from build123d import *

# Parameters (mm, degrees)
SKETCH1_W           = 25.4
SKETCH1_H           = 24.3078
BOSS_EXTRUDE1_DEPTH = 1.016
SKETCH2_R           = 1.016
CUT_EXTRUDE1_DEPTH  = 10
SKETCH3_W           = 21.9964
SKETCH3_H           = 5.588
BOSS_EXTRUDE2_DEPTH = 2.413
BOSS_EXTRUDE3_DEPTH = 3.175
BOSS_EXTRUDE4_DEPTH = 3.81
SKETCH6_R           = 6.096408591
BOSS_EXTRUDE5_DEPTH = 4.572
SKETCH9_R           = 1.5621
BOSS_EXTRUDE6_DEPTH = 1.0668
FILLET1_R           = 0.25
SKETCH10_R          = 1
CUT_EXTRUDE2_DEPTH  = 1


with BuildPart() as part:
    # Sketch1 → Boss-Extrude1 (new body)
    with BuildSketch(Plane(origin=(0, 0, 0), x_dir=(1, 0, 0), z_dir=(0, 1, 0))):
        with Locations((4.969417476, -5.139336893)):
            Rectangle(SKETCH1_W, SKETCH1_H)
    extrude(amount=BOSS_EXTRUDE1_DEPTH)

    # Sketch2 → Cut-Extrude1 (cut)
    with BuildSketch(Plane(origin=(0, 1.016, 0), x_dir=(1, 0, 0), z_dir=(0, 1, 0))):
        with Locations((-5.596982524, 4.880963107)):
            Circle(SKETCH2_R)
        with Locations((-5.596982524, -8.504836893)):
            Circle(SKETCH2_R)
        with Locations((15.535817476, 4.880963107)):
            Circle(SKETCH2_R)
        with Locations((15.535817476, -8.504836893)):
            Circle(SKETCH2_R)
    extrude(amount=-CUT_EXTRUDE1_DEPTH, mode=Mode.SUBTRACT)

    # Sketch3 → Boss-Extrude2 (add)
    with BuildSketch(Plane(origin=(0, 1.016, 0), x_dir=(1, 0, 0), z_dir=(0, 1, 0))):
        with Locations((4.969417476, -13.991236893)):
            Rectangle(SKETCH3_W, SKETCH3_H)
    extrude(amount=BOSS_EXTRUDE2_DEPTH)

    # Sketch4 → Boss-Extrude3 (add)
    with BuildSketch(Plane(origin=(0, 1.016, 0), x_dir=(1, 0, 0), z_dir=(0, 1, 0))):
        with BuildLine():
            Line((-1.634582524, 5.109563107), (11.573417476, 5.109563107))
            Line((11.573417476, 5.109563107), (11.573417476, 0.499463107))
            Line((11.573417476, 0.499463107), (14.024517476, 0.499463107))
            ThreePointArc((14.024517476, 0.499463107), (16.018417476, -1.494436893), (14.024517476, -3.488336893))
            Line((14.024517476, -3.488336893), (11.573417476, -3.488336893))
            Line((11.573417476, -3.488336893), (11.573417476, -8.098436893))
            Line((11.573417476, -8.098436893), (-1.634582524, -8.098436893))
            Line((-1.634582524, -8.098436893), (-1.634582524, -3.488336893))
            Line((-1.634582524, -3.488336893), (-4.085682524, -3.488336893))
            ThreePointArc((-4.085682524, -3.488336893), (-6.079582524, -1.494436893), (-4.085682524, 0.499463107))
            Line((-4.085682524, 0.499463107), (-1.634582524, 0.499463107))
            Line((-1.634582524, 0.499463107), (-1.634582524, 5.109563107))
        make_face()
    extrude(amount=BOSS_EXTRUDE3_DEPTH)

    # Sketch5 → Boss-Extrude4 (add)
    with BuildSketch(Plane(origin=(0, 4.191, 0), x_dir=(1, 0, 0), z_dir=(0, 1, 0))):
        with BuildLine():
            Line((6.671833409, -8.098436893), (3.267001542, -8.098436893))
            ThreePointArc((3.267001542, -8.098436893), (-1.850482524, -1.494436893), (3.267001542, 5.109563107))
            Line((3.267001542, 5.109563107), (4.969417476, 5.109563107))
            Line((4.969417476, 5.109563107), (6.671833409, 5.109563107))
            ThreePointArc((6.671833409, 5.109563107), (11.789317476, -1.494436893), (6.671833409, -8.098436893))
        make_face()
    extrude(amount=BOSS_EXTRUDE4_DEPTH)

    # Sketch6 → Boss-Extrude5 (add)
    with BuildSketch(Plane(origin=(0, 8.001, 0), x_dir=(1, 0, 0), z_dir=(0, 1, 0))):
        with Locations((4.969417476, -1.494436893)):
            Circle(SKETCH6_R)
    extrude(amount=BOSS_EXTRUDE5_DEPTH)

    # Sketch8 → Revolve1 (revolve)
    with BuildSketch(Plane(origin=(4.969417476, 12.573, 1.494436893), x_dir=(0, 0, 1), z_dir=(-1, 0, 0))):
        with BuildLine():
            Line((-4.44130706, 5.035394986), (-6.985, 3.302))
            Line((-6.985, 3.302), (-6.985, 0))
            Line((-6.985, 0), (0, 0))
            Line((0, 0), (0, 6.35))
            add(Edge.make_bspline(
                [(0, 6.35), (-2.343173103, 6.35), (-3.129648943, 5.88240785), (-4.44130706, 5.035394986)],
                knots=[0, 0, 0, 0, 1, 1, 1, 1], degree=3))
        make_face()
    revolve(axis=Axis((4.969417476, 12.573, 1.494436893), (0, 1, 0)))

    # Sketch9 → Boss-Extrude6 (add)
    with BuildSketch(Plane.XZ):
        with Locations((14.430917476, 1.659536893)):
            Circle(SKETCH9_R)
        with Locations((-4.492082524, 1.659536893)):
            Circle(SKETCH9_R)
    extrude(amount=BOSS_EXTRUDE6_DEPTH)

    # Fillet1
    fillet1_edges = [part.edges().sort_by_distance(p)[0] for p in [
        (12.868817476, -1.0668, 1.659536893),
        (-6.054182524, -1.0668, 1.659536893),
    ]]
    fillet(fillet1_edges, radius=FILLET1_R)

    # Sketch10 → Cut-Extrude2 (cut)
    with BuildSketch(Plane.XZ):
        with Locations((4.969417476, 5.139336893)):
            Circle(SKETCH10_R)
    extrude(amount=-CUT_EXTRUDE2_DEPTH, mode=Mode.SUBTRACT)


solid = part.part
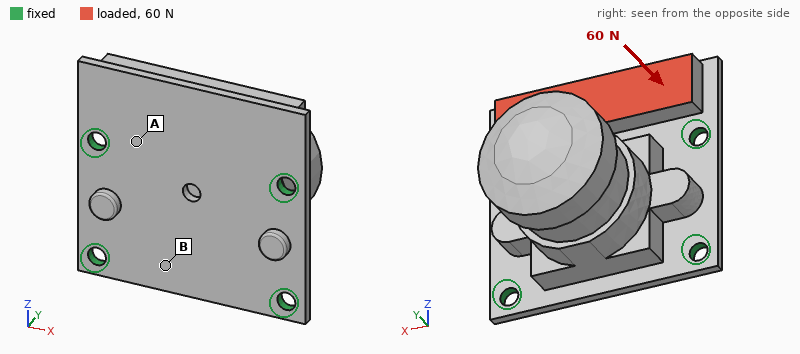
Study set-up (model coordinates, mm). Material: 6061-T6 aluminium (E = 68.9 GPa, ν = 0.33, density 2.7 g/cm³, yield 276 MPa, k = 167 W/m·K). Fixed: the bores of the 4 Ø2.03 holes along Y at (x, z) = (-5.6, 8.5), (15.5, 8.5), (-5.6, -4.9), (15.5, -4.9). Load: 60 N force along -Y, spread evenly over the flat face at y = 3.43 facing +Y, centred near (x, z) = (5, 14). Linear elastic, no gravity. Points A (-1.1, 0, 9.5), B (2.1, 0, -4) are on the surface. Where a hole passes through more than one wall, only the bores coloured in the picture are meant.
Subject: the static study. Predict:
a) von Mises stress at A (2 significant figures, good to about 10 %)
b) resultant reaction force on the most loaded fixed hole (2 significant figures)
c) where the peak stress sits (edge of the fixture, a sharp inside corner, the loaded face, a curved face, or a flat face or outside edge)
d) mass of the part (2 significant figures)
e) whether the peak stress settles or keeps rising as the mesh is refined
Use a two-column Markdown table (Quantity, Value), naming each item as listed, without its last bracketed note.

| Quantity | Value |
|---|---|
| von Mises stress at A | 36 MPa |
| resultant reaction force on the most loaded fixed hole | 41 N |
| where the peak stress sits | edge of the fixture |
| mass of the part | 9.2 g |
| whether the peak stress settles or keeps rising as the mesh is refined | keeps rising |
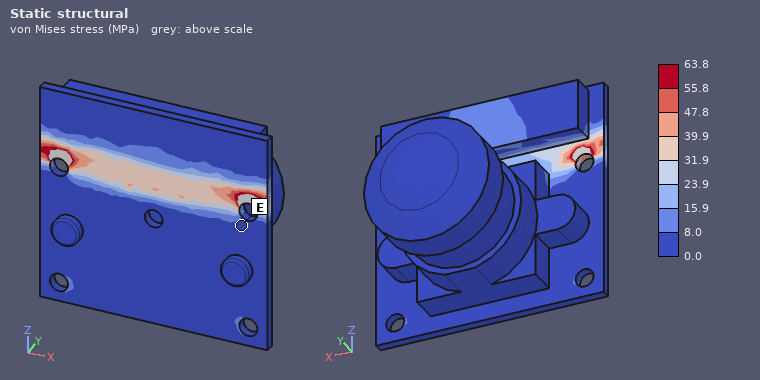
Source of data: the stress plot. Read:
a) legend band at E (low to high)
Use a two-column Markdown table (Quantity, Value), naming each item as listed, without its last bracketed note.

| Quantity | Value |
|---|---|
| legend band at E | 0.0 to 8.0 MPa |
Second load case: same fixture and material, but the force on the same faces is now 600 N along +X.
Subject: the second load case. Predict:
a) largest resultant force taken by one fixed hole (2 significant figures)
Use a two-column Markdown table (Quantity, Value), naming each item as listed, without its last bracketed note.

| Quantity | Value |
|---|---|
| largest resultant force taken by one fixed hole | 310 N |
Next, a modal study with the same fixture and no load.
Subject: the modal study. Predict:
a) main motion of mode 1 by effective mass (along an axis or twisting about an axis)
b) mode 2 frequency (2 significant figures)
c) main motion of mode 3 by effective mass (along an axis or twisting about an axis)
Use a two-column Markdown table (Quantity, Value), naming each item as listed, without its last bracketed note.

| Quantity | Value |
|---|---|
| main motion of mode 1 by effective mass | along Z |
| mode 2 frequency | 7100 Hz |
| main motion of mode 3 by effective mass | along X |
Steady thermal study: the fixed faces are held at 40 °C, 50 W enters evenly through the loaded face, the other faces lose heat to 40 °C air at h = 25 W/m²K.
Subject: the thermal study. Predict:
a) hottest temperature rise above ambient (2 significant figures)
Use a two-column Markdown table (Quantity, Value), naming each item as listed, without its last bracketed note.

| Quantity | Value |
|---|---|
| hottest temperature rise above ambient | 75 K |
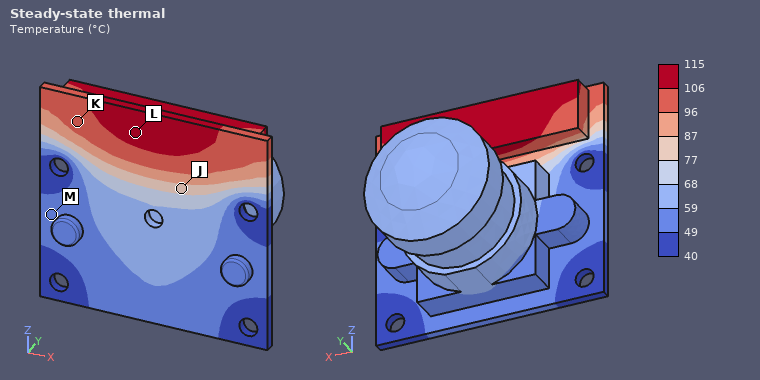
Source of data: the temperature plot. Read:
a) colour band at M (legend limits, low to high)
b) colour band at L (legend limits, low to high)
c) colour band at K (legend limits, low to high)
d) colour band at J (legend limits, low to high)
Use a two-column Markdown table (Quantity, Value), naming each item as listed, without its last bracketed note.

| Quantity | Value |
|---|---|
| colour band at M | 49 to 59 °C |
| colour band at L | 106 to 115 °C |
| colour band at K | 96 to 106 °C |
| colour band at J | 77 to 87 °C |
